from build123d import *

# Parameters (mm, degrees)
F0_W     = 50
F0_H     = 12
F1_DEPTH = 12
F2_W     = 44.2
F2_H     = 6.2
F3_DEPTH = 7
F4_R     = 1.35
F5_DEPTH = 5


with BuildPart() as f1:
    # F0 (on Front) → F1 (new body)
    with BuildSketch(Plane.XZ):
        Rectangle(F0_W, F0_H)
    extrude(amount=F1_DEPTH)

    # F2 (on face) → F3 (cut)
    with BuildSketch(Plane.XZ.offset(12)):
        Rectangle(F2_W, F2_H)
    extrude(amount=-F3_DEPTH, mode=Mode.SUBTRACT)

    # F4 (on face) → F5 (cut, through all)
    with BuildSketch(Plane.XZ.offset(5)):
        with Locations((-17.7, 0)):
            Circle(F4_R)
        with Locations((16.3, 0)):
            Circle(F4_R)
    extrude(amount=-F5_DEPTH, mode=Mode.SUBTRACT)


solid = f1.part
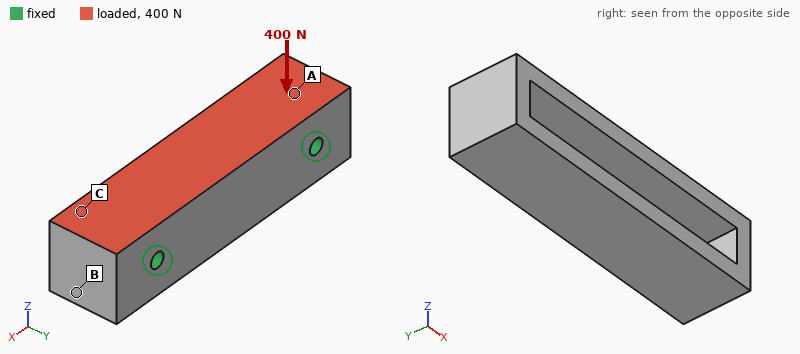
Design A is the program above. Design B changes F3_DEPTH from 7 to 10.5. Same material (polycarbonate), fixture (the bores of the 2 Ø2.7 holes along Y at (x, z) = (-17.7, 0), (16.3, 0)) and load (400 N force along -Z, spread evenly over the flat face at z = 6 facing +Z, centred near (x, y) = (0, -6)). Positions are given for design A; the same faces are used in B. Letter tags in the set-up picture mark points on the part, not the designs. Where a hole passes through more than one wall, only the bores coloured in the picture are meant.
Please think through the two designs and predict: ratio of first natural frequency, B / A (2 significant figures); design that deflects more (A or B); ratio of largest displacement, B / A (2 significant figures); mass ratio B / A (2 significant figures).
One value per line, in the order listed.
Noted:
0.31
B
8.4
0.82
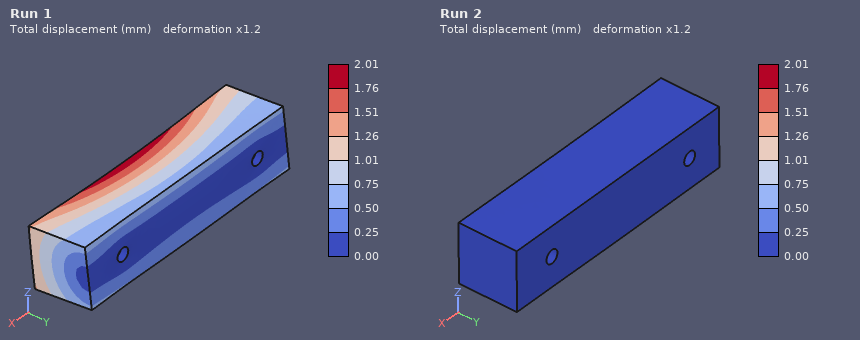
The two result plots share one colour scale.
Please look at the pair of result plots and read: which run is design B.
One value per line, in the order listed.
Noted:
Run 1
